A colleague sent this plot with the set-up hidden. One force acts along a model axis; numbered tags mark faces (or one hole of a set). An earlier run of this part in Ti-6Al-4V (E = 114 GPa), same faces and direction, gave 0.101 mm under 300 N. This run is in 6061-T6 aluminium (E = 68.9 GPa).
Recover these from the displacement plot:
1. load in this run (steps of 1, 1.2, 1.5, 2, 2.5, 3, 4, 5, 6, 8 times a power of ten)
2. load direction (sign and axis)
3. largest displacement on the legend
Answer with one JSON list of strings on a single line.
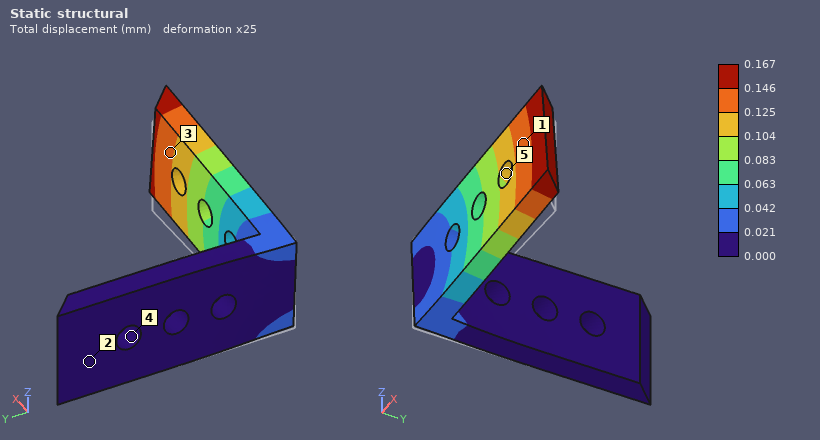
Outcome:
["300 N", "+Z", "0.167 mm"]
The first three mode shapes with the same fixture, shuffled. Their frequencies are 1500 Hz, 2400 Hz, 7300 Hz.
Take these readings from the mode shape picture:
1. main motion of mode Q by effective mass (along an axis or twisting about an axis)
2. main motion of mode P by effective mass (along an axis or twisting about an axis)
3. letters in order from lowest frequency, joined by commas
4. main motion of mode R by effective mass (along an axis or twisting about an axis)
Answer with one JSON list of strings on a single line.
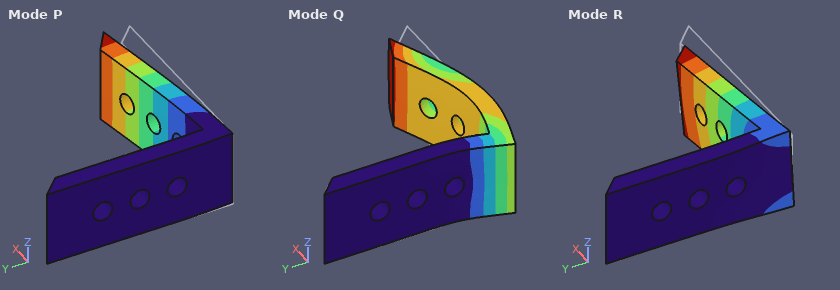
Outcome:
["along X", "along Y", "P, R, Q", "along Z"]
